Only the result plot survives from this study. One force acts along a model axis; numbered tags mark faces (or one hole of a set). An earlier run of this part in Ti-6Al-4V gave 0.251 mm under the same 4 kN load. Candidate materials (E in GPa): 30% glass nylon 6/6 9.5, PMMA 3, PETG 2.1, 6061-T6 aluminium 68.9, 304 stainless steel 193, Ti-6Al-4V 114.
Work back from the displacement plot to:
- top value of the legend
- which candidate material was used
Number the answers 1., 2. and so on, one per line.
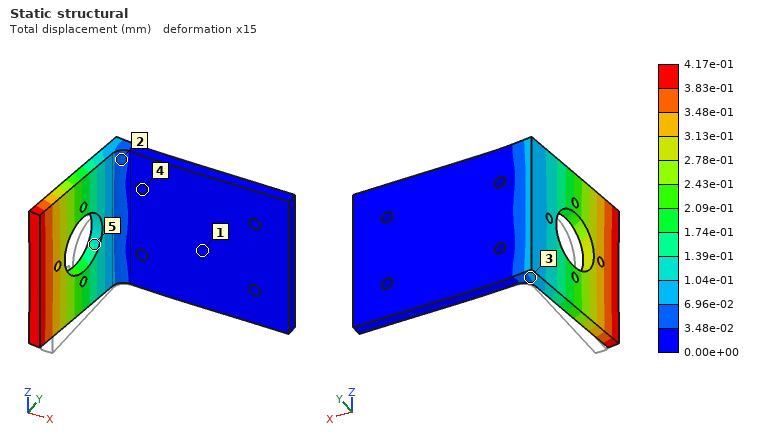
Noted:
1. 4.17e-01 mm
2. 6061-T6 aluminium
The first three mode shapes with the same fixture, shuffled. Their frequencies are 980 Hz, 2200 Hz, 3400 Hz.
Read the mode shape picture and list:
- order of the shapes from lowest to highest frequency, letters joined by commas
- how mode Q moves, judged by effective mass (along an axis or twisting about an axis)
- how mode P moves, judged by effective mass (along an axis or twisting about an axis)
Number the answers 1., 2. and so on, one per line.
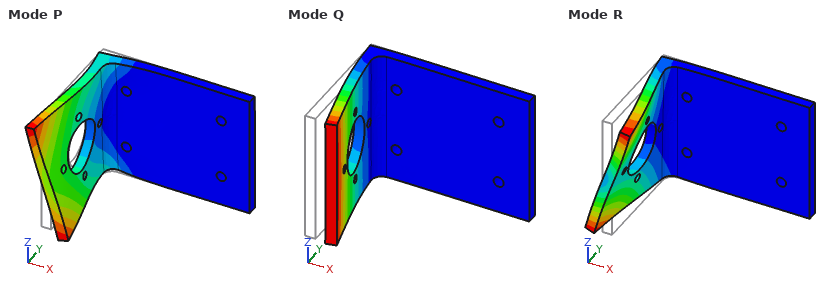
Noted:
1. Q, R, P
2. along X
3. along Z
